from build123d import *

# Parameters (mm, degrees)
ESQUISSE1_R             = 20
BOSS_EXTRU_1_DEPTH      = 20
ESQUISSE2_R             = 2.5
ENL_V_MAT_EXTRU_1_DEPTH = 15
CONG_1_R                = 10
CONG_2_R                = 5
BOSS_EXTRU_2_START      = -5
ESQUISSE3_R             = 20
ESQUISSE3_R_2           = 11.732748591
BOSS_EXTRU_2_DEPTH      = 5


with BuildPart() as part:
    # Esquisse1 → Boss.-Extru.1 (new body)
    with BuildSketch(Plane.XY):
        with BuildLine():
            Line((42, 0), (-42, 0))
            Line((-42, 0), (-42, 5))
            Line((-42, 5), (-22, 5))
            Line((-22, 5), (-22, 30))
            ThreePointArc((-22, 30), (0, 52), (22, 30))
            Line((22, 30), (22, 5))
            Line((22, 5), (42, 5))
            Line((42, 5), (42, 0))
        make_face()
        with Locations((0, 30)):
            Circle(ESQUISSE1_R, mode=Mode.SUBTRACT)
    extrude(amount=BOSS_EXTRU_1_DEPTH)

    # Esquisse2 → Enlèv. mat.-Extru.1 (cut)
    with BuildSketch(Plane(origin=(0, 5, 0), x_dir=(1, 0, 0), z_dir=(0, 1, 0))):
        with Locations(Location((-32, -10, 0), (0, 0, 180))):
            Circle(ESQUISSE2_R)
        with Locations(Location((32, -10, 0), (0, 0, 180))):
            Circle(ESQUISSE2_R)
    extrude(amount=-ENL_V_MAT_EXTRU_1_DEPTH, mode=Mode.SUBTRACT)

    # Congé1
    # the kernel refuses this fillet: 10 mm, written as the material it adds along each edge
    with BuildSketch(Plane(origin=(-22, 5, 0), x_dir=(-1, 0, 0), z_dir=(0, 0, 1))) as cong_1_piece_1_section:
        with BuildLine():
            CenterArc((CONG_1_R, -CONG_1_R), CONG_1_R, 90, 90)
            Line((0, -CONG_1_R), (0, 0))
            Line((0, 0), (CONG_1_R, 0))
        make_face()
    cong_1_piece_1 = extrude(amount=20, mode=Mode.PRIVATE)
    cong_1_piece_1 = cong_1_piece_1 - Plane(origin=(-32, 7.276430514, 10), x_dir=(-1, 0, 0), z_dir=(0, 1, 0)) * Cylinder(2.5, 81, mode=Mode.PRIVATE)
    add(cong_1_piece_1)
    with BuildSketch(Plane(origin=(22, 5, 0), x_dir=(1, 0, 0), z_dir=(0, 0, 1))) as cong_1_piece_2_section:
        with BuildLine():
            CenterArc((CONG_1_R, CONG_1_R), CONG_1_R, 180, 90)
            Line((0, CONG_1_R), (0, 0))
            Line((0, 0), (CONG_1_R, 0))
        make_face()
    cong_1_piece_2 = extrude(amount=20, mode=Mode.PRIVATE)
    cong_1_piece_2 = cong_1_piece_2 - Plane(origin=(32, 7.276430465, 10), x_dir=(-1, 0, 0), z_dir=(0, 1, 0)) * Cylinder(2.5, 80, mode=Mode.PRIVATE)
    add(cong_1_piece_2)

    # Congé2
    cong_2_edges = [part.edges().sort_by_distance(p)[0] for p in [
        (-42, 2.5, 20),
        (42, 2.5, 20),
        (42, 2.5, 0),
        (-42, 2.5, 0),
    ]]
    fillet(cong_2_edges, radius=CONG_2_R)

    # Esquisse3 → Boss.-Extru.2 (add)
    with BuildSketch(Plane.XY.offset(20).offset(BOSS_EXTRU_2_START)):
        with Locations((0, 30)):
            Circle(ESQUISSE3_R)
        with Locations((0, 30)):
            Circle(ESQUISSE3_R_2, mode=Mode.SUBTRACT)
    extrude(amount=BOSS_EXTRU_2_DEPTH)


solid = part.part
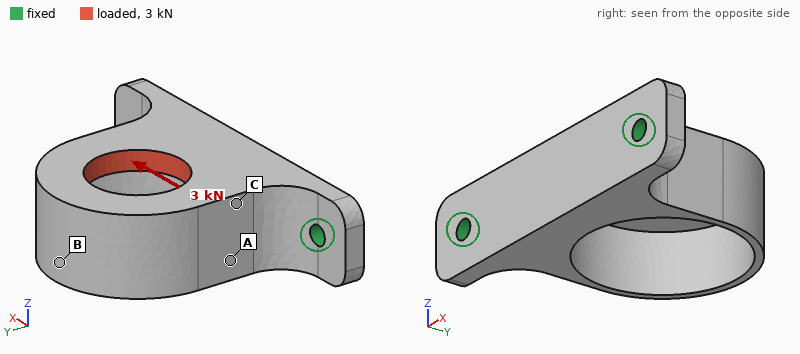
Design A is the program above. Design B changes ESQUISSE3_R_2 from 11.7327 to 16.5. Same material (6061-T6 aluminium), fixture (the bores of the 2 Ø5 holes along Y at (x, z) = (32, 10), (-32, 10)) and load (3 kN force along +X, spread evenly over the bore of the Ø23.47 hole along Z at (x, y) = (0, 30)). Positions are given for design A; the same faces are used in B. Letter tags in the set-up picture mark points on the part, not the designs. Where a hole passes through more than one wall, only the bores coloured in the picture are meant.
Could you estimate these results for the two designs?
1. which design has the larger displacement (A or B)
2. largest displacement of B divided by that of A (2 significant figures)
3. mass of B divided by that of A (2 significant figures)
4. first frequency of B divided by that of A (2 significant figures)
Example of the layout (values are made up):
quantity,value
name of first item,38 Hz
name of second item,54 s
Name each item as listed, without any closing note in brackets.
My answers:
quantity,value
which design has the larger displacement,B
largest displacement of B divided by that of A,2.4
mass of B divided by that of A,0.92
first frequency of B divided by that of A,1.1
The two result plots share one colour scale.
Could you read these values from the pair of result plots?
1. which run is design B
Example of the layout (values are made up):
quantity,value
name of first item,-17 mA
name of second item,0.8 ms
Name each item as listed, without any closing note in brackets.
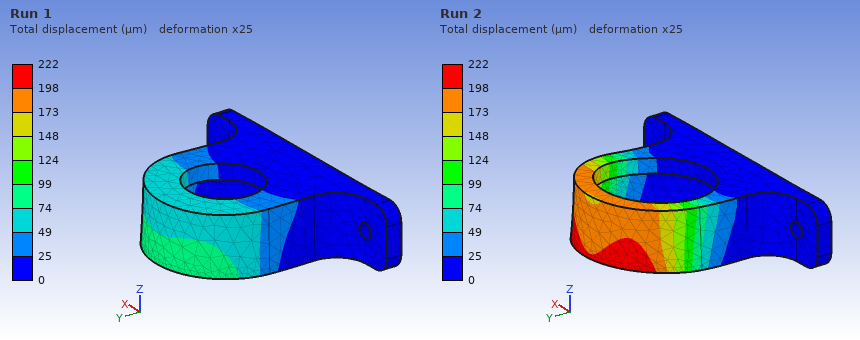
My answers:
quantity,value
which run is design B,Run 2
